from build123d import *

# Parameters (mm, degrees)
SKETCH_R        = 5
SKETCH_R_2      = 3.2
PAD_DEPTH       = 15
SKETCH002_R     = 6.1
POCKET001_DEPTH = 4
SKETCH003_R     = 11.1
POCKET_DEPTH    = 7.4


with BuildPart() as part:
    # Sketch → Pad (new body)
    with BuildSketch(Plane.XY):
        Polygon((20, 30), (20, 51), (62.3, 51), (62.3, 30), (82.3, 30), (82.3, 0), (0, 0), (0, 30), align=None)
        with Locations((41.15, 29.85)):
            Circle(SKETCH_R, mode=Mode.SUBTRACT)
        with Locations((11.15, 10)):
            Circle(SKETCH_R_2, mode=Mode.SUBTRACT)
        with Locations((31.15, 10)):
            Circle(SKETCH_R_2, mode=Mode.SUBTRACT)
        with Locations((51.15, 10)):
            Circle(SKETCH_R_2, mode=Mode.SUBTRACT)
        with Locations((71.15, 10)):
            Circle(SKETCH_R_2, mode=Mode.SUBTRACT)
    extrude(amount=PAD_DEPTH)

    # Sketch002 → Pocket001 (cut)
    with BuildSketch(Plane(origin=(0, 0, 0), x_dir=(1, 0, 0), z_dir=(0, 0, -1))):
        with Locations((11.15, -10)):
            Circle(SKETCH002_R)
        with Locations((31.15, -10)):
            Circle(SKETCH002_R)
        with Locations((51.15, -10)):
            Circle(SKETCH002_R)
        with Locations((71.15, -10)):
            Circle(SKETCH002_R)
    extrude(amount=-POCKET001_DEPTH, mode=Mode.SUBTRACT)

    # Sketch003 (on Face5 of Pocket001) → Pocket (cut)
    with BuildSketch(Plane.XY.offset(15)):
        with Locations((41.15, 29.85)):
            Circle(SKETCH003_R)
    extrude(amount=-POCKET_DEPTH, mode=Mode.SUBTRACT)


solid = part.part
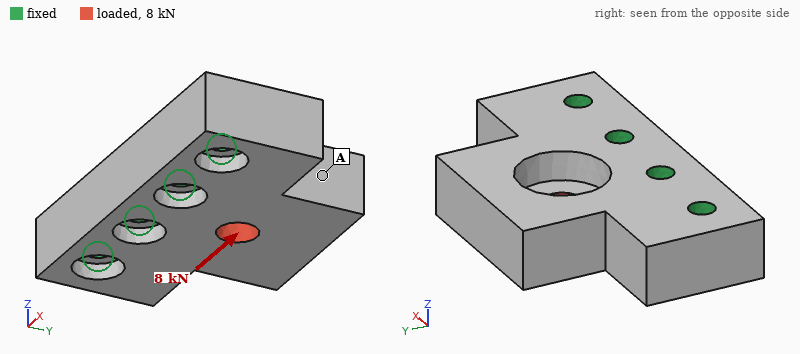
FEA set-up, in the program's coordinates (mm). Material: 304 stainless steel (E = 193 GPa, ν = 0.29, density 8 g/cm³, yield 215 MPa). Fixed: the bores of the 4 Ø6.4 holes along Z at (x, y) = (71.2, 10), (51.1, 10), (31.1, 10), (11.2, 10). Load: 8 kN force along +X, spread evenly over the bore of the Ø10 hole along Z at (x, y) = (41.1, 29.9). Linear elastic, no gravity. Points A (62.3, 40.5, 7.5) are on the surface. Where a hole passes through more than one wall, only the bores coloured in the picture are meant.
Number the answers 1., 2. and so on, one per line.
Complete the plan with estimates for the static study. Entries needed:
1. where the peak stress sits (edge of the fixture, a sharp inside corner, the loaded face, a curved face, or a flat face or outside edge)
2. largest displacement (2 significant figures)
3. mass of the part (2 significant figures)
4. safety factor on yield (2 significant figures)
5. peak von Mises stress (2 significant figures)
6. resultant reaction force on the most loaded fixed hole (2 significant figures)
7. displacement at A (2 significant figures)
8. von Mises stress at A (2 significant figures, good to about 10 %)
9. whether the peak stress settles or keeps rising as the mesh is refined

1. the loaded face
2. 5.7 µm
3. 350 g
4. 3.2
5. 66 MPa
6. 3.0 kN
7. 4.1 µm
8. 7.4 MPa
9. settles
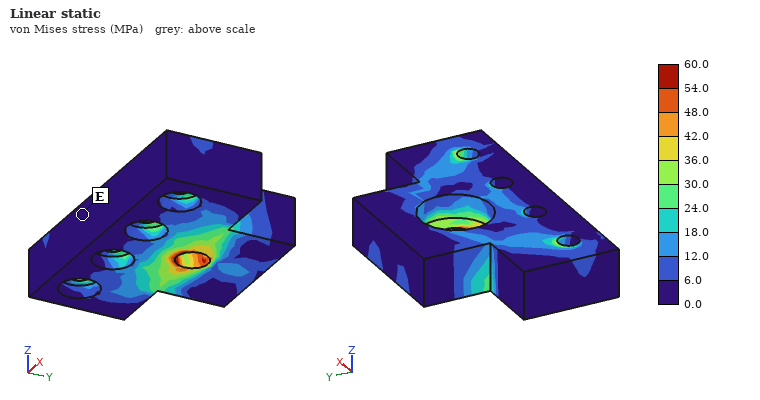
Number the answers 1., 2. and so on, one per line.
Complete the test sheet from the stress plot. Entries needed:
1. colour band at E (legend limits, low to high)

1. 0.0 to 6.0 MPa
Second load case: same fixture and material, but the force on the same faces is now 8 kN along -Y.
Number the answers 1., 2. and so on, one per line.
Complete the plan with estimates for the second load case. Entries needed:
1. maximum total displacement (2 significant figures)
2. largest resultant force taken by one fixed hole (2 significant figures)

1. 11 µm
2. 3.1 kN
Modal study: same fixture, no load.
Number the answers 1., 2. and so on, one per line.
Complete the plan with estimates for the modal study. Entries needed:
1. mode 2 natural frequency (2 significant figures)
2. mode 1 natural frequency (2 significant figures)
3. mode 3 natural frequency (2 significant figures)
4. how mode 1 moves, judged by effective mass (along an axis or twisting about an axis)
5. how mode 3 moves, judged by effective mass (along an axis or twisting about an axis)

1. 12 kHz
2. 6100 Hz
3. 16 kHz
4. along Z
5. along X
